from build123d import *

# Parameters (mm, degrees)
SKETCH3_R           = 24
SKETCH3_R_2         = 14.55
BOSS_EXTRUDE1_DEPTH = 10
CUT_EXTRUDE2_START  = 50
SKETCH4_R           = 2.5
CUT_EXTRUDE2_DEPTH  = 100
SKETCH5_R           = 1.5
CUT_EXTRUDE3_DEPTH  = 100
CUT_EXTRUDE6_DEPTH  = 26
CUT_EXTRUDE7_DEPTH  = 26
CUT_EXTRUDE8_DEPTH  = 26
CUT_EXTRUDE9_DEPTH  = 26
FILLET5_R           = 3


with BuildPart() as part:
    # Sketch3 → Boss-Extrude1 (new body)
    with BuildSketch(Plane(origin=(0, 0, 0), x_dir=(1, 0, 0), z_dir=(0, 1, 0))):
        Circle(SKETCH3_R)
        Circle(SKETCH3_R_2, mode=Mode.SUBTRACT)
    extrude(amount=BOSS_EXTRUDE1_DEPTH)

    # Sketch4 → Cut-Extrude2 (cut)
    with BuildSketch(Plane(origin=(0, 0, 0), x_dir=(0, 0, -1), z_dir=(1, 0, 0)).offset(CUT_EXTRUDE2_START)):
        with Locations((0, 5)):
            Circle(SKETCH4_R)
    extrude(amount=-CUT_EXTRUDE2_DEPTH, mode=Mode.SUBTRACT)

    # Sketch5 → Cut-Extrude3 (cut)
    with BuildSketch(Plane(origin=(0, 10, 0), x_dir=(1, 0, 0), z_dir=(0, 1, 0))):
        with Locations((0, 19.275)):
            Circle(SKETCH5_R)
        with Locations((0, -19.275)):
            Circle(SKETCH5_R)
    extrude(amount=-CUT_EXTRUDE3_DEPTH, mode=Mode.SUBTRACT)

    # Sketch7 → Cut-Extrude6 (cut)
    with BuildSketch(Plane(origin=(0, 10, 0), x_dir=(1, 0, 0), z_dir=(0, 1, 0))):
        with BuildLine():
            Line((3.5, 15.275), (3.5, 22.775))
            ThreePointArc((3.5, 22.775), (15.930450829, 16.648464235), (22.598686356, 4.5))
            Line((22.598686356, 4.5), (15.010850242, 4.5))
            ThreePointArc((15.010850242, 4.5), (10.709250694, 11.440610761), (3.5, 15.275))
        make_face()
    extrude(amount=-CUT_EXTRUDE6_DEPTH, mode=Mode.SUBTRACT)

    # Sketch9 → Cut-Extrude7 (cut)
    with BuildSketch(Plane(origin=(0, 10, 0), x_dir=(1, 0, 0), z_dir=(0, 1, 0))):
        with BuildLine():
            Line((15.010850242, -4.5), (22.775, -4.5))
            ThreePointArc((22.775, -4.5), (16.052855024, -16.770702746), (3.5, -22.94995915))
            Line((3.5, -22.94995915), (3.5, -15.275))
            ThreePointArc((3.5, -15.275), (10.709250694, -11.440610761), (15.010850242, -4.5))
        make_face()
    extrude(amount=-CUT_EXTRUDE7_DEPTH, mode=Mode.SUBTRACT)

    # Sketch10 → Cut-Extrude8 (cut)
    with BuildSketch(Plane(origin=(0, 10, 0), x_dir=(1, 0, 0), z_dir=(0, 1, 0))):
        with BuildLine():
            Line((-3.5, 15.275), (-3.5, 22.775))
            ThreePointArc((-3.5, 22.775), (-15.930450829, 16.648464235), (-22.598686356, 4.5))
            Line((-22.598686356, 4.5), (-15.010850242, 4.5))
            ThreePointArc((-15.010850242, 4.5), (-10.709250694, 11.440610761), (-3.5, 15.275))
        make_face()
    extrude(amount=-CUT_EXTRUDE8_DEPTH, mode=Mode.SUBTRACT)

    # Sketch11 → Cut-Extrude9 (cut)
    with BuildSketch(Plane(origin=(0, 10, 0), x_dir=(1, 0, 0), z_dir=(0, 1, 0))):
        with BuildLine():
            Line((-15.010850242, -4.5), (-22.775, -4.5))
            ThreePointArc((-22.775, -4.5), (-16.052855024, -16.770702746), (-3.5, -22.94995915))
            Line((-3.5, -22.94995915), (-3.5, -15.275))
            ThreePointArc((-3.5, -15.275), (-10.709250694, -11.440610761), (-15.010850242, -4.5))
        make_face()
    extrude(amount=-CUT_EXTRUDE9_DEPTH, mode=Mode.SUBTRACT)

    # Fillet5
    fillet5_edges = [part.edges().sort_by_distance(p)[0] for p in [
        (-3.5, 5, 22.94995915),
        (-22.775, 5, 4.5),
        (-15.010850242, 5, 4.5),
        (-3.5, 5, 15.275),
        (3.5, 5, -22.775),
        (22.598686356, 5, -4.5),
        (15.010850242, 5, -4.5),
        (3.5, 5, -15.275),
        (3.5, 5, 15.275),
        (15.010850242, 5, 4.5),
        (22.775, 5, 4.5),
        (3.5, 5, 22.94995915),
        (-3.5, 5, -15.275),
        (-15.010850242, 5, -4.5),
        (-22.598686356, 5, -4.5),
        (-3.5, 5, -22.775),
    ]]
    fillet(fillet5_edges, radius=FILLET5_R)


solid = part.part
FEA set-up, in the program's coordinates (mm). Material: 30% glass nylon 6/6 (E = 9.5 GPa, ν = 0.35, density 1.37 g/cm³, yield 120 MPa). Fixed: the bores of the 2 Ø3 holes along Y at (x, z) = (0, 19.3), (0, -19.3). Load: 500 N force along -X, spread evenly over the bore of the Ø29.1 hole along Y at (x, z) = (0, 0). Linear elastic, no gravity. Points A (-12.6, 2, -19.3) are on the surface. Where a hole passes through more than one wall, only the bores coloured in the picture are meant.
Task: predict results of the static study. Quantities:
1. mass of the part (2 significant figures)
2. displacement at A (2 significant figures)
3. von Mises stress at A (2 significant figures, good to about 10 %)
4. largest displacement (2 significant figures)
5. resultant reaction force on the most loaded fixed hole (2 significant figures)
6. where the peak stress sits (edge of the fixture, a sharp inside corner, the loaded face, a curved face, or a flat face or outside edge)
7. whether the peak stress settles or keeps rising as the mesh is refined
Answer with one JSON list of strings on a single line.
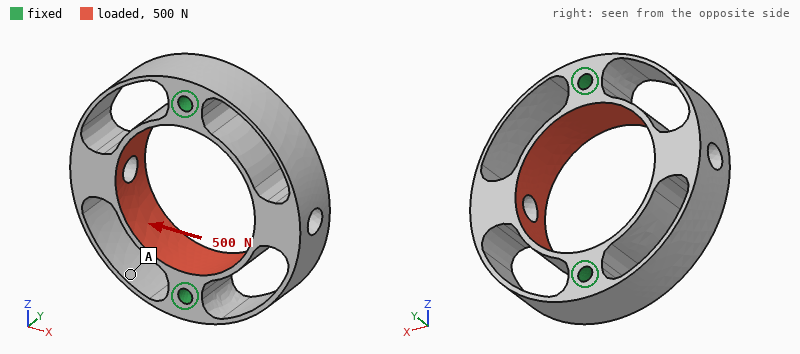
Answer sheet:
["6.3 g", "16 µm", "2.8 MPa", "29 µm", "250 N", "edge of the fixture", "keeps rising"]
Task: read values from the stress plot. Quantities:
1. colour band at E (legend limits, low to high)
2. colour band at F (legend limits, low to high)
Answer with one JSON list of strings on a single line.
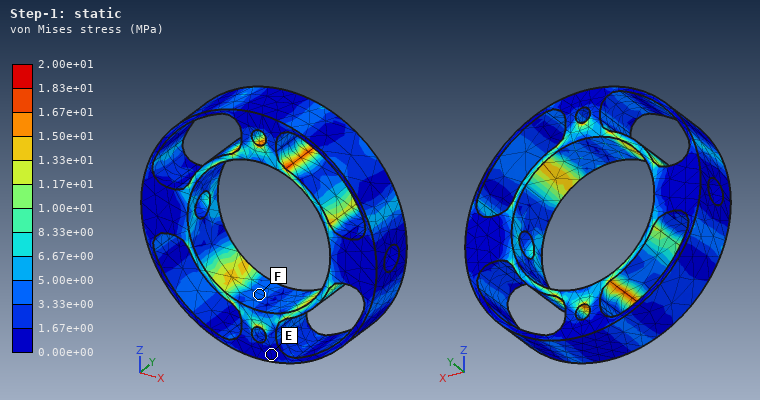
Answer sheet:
["0.00e+00 to 1.67e+00 MPa", "3.33e+00 to 5.00e+00 MPa"]
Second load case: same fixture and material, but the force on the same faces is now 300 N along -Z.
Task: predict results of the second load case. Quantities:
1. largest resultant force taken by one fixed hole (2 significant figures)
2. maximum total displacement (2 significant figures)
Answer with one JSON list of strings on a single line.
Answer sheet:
["150 N", "0.20 mm"]
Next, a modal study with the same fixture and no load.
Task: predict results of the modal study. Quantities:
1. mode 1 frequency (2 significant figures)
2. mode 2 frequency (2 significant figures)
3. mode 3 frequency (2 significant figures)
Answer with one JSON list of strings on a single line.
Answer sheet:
["2700 Hz", "2800 Hz", "4000 Hz"]
